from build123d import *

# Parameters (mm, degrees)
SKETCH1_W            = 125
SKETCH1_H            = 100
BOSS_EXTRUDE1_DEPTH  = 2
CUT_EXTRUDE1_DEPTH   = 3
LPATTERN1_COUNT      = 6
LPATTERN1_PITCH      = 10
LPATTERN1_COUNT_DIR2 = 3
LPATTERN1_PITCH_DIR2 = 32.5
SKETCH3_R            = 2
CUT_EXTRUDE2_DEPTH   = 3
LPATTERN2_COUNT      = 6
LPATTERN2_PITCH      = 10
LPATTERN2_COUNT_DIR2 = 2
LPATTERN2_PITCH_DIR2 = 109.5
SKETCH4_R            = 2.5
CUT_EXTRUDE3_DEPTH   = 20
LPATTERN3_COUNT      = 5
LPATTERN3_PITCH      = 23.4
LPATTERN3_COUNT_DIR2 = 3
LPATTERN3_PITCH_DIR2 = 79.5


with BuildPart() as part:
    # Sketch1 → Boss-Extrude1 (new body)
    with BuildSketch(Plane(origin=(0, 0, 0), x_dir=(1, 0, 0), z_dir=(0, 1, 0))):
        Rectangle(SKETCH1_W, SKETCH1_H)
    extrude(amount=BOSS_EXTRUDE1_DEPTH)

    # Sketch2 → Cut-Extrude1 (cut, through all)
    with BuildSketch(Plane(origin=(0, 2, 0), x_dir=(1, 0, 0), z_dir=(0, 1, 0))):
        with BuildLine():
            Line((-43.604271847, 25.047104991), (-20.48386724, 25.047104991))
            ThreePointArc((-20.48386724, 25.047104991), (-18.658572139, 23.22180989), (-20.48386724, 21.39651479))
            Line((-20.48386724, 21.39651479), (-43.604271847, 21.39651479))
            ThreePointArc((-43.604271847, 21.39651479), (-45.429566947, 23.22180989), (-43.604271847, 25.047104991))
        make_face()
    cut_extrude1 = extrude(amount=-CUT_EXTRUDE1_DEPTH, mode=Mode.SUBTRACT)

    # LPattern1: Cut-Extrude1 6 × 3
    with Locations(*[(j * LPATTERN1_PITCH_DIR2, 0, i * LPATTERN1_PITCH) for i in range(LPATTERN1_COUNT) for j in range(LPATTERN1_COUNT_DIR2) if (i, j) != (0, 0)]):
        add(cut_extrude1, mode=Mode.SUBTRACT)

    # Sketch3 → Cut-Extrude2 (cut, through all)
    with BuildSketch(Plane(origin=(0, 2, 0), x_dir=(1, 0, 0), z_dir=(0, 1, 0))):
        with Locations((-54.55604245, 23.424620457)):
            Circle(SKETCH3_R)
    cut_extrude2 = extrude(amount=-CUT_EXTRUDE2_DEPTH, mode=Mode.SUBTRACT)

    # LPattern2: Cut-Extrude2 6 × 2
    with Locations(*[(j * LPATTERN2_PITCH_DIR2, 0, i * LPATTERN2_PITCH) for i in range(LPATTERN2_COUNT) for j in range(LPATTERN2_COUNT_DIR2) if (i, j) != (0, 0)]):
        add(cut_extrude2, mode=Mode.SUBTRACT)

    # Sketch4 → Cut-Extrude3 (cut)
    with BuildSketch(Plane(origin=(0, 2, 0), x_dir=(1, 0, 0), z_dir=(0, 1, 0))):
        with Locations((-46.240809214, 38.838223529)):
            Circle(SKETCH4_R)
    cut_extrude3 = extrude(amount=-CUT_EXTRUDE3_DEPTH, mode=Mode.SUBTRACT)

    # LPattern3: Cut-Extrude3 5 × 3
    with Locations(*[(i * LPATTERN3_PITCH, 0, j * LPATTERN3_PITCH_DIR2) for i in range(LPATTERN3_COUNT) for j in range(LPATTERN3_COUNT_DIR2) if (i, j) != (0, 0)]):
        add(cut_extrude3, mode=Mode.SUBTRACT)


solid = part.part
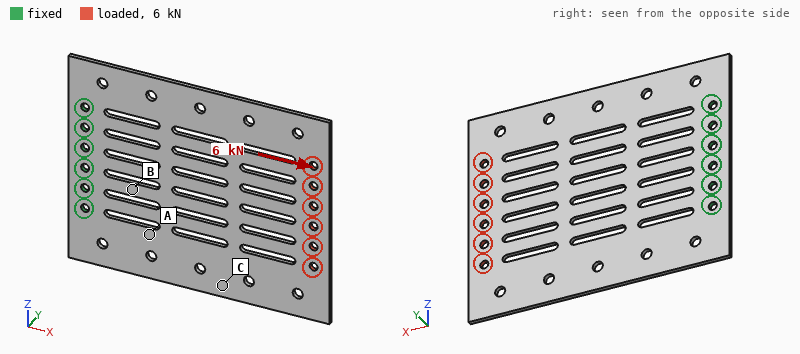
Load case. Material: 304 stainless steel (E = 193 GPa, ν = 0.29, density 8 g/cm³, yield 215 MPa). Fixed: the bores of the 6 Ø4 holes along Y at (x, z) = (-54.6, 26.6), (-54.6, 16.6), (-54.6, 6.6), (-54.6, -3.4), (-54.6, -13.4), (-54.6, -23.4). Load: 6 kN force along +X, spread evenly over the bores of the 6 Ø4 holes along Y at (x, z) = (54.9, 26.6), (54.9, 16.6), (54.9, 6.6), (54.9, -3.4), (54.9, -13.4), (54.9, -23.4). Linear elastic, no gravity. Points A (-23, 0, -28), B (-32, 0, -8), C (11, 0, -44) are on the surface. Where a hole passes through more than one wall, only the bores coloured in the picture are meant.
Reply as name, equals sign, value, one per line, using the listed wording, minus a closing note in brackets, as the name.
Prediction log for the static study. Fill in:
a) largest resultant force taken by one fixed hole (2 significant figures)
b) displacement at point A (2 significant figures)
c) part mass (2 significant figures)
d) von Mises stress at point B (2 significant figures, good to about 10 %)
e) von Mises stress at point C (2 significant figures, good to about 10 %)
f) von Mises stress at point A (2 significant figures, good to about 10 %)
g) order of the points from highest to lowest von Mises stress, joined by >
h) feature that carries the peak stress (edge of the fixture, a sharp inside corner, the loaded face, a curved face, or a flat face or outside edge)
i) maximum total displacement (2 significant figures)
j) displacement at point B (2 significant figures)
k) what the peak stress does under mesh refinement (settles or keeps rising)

largest resultant force taken by one fixed hole = 1.7 kN
displacement at point A = 11 µm
part mass = 170 g
von Mises stress at point B = 62 MPa
von Mises stress at point C = 14 MPa
von Mises stress at point A = 35 MPa
order of the points from highest to lowest von Mises stress, joined by > = B > A > C
feature that carries the peak stress = edge of the fixture
maximum total displacement = 37 µm
displacement at point B = 6.3 µm
what the peak stress does under mesh refinement = keeps rising
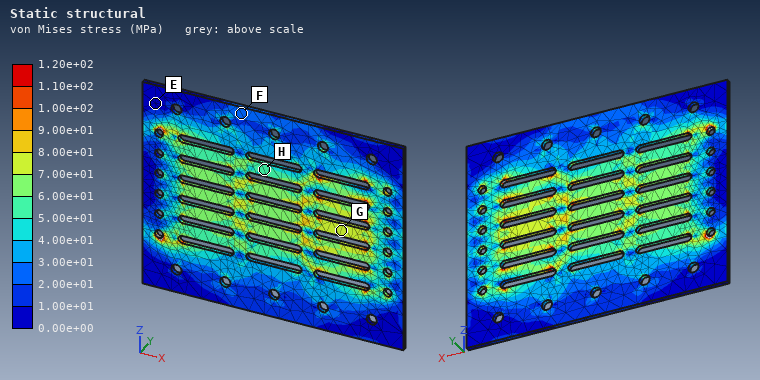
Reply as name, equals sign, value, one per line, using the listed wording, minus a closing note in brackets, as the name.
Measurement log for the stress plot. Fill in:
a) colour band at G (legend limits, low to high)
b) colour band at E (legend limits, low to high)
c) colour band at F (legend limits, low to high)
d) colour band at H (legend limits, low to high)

colour band at G = 7.00e+01 to 8.00e+01 MPa
colour band at E = 0.00e+00 to 1.00e+01 MPa
colour band at F = 2.00e+01 to 3.00e+01 MPa
colour band at H = 5.00e+01 to 6.00e+01 MPa
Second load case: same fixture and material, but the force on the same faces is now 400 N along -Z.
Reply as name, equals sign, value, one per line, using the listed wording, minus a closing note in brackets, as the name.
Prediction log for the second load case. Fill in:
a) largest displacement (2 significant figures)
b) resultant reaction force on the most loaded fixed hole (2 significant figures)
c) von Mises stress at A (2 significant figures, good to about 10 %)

largest displacement = 62 µm
resultant reaction force on the most loaded fixed hole = 840 N
von Mises stress at A = 13 MPa
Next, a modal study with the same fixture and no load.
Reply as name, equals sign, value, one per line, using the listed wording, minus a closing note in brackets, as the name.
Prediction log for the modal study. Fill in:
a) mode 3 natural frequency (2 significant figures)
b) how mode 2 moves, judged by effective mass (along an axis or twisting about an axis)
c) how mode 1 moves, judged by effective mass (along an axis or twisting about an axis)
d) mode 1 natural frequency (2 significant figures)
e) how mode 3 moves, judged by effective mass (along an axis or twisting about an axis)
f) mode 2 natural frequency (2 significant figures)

mode 3 natural frequency = 670 Hz
how mode 2 moves, judged by effective mass = twisting about X
how mode 1 moves, judged by effective mass = along Y
mode 1 natural frequency = 110 Hz
how mode 3 moves, judged by effective mass = along Y
mode 2 natural frequency = 270 Hz
